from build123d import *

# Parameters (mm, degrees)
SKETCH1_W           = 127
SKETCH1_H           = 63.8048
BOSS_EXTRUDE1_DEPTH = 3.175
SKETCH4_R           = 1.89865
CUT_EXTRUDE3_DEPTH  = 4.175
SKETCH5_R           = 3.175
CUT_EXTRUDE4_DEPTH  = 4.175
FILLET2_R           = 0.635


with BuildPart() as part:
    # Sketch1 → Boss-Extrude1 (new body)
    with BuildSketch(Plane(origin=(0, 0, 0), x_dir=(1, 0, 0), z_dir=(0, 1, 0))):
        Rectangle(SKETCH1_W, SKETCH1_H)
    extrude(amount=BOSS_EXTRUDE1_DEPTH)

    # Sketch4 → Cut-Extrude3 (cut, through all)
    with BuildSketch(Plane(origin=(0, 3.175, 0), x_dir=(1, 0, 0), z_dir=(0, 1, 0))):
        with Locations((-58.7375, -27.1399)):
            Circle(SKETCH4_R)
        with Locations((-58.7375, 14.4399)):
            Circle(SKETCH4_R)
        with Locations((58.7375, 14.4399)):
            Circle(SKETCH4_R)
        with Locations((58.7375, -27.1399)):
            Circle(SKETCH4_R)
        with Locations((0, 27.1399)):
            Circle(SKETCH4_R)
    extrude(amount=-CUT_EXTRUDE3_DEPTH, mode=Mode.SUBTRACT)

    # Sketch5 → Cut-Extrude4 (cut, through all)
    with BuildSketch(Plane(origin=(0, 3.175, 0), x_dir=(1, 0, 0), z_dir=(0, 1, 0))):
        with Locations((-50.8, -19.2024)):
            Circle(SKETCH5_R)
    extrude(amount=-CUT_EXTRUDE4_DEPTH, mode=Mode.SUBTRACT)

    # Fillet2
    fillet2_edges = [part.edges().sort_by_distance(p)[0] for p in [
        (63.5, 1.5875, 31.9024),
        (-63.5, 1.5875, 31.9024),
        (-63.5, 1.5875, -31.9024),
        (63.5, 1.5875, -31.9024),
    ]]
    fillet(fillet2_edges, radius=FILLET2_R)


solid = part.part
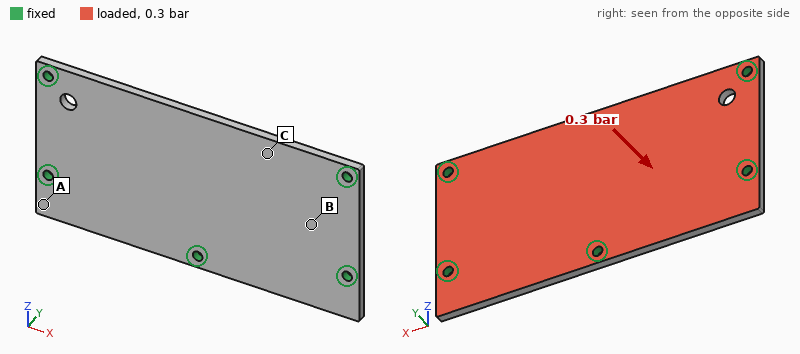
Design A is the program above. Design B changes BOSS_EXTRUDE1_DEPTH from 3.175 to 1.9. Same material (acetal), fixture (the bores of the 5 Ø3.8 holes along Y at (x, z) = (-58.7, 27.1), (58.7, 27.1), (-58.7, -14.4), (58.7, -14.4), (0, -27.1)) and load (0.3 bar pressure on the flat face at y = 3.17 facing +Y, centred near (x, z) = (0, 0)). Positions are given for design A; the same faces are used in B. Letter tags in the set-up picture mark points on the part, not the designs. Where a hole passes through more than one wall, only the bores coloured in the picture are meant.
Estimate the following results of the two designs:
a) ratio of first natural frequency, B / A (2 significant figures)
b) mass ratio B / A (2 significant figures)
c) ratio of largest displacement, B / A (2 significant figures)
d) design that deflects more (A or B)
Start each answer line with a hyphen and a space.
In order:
- 0.61
- 0.60
- 4.4
- B
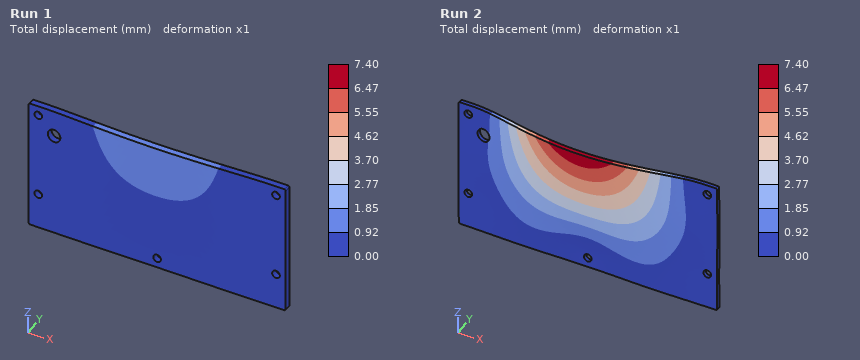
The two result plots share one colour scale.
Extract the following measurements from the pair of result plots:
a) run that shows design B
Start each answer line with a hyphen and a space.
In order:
- Run 2
